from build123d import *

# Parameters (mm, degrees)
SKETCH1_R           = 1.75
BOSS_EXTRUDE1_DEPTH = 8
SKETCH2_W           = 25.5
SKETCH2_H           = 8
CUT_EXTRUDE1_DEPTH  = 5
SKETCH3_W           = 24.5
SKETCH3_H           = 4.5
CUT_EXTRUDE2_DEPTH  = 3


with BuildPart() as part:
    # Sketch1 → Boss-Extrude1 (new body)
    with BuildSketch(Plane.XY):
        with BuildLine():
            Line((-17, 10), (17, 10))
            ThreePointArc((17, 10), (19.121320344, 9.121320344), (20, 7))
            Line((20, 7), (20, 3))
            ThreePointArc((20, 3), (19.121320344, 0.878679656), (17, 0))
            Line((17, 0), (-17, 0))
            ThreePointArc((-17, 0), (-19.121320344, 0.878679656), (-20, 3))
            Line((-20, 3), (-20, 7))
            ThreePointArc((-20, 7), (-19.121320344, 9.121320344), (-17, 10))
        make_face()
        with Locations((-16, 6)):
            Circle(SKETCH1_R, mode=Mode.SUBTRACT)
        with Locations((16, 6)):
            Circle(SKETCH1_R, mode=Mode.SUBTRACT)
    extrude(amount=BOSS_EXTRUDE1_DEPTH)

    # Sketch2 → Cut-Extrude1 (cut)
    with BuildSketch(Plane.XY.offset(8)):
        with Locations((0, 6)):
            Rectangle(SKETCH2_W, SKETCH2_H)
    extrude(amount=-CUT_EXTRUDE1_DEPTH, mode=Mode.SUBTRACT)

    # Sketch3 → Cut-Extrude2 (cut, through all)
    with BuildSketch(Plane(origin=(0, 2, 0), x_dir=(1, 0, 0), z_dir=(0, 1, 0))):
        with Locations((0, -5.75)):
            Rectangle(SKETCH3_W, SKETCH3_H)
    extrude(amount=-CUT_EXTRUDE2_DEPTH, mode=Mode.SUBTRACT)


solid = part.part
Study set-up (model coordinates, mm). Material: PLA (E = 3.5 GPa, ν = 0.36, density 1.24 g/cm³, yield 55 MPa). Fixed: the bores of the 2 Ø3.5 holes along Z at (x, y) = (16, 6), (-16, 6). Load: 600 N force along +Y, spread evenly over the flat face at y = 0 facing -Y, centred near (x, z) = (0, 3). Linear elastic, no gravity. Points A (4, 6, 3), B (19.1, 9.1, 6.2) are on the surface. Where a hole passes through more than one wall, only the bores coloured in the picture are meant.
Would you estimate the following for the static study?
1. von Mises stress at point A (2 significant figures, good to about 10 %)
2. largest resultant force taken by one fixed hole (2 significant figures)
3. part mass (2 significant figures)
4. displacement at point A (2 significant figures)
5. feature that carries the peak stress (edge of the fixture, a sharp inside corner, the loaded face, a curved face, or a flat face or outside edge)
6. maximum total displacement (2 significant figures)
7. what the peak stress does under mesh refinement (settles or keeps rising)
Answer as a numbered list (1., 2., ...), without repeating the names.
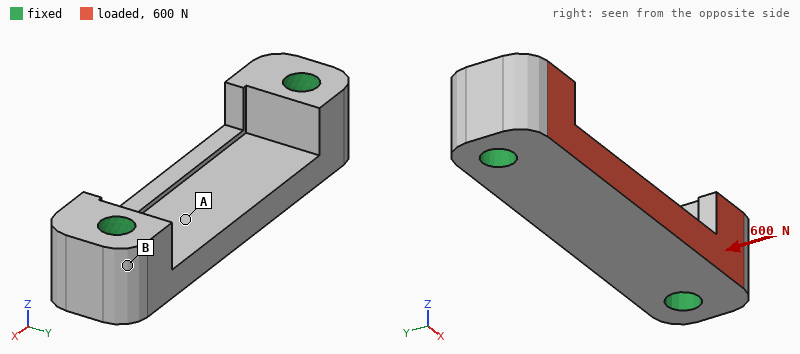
1. 5.8 MPa
2. 300 N
3. 2.2 g
4. 0.085 mm
5. edge of the fixture
6. 0.10 mm
7. keeps rising
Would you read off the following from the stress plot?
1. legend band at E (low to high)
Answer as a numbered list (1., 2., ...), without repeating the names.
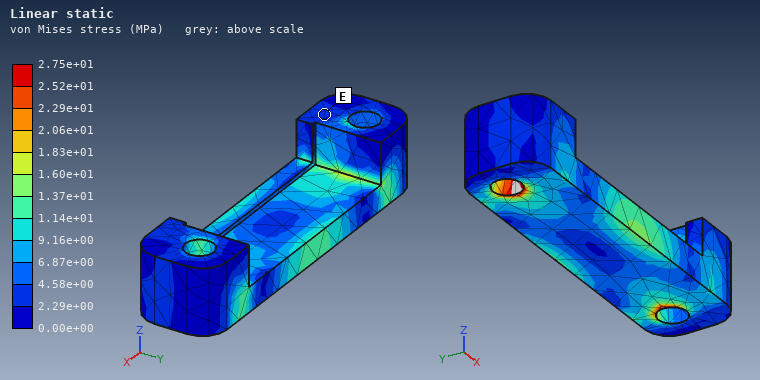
1. 2.29e+00 to 4.58e+00 MPa
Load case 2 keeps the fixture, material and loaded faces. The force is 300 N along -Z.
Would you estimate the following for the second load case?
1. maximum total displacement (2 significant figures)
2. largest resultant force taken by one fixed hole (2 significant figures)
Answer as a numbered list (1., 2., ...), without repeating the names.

1. 0.27 mm
2. 150 N
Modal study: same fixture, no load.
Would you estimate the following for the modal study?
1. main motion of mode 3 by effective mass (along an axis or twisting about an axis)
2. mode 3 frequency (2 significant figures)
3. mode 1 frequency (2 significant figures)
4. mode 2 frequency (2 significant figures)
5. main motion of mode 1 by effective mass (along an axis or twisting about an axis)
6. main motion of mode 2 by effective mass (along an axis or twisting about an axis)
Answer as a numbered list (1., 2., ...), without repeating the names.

1. along Y
2. 11 kHz
3. 6400 Hz
4. 11 kHz
5. along Z
6. along Y
